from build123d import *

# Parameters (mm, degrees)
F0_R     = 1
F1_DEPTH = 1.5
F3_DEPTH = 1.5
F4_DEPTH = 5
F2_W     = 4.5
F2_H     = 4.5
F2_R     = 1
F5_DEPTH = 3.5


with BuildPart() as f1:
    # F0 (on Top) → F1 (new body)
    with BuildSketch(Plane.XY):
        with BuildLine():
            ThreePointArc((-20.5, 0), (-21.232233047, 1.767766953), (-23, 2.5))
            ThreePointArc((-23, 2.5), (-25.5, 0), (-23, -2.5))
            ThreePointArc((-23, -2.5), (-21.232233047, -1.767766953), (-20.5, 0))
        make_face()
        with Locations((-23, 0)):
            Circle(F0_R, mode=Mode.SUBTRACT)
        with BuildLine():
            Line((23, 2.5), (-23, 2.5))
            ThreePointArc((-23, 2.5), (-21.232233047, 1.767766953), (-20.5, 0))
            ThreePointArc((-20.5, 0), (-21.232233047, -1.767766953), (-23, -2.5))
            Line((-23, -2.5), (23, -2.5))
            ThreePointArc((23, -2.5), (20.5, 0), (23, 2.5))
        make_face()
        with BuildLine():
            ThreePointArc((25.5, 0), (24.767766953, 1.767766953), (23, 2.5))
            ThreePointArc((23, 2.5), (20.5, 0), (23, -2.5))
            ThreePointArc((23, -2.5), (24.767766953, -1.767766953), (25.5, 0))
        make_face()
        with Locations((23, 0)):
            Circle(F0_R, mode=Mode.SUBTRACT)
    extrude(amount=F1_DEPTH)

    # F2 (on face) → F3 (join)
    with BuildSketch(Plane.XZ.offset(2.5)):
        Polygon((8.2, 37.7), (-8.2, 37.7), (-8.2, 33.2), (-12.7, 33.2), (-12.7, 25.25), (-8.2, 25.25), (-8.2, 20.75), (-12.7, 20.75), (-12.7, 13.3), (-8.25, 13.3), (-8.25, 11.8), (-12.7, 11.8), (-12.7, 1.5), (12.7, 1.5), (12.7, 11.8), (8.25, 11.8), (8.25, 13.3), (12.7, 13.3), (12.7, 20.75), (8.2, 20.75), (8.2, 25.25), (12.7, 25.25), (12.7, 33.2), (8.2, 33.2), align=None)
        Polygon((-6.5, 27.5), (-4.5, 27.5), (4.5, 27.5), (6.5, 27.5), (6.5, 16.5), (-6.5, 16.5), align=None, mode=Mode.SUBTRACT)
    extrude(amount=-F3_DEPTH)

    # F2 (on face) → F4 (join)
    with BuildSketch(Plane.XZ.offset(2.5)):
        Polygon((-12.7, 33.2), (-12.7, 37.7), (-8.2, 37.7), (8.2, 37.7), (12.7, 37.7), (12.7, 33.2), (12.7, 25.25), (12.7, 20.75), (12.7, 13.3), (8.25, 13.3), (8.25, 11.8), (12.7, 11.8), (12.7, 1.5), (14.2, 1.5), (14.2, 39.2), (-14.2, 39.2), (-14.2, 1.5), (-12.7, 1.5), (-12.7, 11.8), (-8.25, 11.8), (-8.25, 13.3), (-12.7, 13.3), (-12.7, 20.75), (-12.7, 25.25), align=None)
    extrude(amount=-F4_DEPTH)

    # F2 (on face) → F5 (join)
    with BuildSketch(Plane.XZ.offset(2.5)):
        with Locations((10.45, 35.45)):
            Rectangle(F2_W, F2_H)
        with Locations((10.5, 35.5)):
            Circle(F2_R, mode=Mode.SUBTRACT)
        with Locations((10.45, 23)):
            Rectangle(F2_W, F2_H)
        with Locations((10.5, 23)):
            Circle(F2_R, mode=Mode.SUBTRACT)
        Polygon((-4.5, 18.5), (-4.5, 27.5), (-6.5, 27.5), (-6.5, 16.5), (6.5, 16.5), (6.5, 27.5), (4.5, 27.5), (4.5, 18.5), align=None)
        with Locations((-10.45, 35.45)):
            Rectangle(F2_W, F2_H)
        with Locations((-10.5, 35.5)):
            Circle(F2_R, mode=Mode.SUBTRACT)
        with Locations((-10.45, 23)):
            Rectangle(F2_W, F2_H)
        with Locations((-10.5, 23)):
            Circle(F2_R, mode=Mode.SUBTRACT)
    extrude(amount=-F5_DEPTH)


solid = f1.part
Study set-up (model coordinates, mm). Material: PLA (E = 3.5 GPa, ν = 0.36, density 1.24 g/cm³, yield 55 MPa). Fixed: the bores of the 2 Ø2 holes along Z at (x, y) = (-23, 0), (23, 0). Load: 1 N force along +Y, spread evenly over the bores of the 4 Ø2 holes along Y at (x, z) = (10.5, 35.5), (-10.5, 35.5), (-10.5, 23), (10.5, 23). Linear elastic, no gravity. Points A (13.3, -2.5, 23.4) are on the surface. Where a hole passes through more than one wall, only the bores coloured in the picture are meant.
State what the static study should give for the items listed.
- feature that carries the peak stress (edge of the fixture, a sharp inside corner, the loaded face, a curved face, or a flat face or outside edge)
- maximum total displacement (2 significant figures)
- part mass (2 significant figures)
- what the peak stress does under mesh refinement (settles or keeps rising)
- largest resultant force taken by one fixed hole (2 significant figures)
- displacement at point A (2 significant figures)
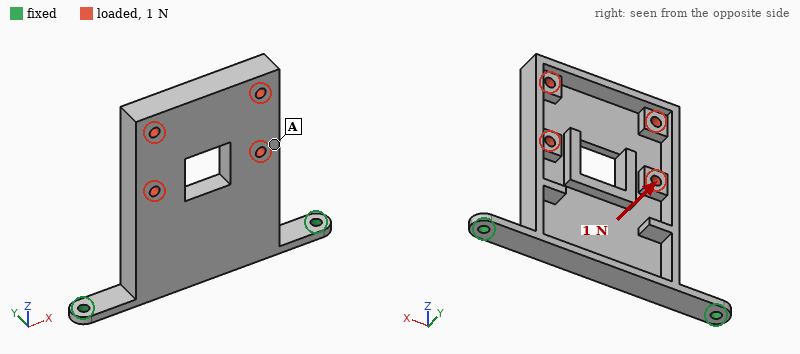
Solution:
edge of the fixture
0.75 mm
3.3 g
keeps rising
0.63 N
0.44 mm
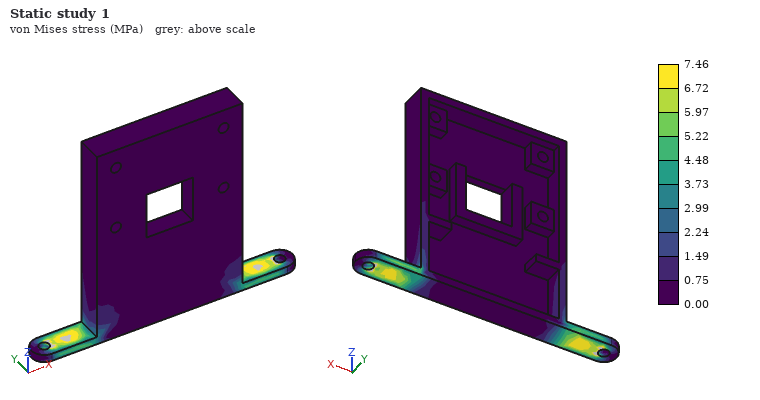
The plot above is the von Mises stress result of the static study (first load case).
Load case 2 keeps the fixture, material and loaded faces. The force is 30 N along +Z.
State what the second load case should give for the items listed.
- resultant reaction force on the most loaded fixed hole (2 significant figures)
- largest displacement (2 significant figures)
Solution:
17 N
0.60 mm
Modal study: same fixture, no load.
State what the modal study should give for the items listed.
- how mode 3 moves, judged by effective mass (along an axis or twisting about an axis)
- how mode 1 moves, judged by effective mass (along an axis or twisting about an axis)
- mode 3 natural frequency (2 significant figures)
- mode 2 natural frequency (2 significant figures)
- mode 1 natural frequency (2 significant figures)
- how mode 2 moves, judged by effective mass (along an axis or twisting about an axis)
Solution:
along X
along Y
850 Hz
700 Hz
150 Hz
along X
